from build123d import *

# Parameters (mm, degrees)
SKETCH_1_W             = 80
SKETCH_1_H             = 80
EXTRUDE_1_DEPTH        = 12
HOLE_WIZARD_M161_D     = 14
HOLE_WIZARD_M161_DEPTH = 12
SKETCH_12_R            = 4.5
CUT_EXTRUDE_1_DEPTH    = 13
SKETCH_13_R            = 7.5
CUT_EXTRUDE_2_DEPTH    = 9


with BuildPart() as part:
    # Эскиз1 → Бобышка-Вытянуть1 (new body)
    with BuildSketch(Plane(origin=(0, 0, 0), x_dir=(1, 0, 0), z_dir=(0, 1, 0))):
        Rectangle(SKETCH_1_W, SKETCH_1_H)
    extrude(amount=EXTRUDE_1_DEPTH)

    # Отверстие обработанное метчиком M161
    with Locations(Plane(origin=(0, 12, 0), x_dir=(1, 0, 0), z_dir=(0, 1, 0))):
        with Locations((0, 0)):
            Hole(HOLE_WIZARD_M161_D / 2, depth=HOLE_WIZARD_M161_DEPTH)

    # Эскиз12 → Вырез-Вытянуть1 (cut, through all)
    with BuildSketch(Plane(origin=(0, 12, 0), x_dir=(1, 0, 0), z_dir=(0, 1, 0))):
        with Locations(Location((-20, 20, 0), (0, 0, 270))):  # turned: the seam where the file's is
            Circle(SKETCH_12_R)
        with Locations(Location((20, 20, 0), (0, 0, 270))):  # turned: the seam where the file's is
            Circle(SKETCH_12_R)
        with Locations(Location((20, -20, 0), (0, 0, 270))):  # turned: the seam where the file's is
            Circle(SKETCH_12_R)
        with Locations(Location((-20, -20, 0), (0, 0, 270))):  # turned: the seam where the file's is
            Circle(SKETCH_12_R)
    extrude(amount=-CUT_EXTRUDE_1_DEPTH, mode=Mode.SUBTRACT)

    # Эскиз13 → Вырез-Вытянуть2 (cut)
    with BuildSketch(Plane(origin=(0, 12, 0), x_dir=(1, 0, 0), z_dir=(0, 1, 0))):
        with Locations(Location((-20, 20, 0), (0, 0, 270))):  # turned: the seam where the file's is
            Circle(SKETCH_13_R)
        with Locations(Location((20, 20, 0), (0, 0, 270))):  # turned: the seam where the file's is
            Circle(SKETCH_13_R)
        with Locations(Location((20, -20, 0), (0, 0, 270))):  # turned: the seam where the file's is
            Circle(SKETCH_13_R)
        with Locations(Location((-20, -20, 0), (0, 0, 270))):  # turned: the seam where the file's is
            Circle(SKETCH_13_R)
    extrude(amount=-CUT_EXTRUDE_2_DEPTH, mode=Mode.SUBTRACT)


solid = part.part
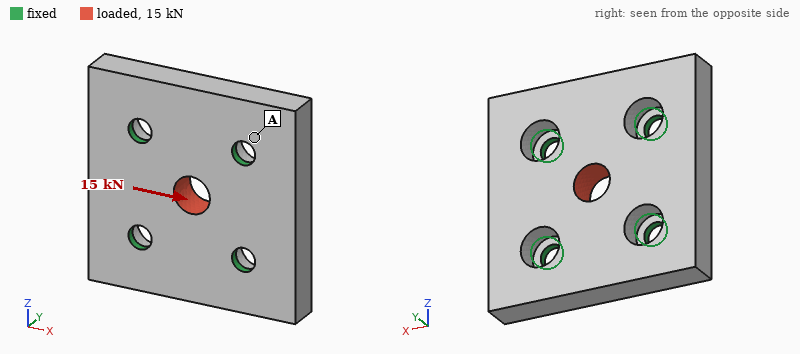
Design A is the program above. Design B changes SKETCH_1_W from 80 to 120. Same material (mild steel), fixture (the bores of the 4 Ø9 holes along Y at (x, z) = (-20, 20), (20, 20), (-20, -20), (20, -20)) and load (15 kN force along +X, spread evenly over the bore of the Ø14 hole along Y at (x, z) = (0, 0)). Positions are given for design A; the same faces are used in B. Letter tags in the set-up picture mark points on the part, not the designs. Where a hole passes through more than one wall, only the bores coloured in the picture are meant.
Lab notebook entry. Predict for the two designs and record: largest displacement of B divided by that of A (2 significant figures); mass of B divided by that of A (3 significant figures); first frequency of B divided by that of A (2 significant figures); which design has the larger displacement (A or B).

1.4
1.57
0.39
B
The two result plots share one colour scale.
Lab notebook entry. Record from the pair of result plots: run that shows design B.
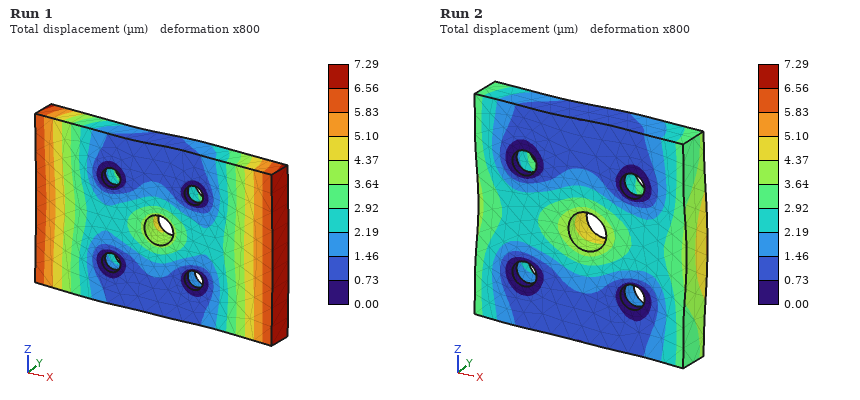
Run 1
